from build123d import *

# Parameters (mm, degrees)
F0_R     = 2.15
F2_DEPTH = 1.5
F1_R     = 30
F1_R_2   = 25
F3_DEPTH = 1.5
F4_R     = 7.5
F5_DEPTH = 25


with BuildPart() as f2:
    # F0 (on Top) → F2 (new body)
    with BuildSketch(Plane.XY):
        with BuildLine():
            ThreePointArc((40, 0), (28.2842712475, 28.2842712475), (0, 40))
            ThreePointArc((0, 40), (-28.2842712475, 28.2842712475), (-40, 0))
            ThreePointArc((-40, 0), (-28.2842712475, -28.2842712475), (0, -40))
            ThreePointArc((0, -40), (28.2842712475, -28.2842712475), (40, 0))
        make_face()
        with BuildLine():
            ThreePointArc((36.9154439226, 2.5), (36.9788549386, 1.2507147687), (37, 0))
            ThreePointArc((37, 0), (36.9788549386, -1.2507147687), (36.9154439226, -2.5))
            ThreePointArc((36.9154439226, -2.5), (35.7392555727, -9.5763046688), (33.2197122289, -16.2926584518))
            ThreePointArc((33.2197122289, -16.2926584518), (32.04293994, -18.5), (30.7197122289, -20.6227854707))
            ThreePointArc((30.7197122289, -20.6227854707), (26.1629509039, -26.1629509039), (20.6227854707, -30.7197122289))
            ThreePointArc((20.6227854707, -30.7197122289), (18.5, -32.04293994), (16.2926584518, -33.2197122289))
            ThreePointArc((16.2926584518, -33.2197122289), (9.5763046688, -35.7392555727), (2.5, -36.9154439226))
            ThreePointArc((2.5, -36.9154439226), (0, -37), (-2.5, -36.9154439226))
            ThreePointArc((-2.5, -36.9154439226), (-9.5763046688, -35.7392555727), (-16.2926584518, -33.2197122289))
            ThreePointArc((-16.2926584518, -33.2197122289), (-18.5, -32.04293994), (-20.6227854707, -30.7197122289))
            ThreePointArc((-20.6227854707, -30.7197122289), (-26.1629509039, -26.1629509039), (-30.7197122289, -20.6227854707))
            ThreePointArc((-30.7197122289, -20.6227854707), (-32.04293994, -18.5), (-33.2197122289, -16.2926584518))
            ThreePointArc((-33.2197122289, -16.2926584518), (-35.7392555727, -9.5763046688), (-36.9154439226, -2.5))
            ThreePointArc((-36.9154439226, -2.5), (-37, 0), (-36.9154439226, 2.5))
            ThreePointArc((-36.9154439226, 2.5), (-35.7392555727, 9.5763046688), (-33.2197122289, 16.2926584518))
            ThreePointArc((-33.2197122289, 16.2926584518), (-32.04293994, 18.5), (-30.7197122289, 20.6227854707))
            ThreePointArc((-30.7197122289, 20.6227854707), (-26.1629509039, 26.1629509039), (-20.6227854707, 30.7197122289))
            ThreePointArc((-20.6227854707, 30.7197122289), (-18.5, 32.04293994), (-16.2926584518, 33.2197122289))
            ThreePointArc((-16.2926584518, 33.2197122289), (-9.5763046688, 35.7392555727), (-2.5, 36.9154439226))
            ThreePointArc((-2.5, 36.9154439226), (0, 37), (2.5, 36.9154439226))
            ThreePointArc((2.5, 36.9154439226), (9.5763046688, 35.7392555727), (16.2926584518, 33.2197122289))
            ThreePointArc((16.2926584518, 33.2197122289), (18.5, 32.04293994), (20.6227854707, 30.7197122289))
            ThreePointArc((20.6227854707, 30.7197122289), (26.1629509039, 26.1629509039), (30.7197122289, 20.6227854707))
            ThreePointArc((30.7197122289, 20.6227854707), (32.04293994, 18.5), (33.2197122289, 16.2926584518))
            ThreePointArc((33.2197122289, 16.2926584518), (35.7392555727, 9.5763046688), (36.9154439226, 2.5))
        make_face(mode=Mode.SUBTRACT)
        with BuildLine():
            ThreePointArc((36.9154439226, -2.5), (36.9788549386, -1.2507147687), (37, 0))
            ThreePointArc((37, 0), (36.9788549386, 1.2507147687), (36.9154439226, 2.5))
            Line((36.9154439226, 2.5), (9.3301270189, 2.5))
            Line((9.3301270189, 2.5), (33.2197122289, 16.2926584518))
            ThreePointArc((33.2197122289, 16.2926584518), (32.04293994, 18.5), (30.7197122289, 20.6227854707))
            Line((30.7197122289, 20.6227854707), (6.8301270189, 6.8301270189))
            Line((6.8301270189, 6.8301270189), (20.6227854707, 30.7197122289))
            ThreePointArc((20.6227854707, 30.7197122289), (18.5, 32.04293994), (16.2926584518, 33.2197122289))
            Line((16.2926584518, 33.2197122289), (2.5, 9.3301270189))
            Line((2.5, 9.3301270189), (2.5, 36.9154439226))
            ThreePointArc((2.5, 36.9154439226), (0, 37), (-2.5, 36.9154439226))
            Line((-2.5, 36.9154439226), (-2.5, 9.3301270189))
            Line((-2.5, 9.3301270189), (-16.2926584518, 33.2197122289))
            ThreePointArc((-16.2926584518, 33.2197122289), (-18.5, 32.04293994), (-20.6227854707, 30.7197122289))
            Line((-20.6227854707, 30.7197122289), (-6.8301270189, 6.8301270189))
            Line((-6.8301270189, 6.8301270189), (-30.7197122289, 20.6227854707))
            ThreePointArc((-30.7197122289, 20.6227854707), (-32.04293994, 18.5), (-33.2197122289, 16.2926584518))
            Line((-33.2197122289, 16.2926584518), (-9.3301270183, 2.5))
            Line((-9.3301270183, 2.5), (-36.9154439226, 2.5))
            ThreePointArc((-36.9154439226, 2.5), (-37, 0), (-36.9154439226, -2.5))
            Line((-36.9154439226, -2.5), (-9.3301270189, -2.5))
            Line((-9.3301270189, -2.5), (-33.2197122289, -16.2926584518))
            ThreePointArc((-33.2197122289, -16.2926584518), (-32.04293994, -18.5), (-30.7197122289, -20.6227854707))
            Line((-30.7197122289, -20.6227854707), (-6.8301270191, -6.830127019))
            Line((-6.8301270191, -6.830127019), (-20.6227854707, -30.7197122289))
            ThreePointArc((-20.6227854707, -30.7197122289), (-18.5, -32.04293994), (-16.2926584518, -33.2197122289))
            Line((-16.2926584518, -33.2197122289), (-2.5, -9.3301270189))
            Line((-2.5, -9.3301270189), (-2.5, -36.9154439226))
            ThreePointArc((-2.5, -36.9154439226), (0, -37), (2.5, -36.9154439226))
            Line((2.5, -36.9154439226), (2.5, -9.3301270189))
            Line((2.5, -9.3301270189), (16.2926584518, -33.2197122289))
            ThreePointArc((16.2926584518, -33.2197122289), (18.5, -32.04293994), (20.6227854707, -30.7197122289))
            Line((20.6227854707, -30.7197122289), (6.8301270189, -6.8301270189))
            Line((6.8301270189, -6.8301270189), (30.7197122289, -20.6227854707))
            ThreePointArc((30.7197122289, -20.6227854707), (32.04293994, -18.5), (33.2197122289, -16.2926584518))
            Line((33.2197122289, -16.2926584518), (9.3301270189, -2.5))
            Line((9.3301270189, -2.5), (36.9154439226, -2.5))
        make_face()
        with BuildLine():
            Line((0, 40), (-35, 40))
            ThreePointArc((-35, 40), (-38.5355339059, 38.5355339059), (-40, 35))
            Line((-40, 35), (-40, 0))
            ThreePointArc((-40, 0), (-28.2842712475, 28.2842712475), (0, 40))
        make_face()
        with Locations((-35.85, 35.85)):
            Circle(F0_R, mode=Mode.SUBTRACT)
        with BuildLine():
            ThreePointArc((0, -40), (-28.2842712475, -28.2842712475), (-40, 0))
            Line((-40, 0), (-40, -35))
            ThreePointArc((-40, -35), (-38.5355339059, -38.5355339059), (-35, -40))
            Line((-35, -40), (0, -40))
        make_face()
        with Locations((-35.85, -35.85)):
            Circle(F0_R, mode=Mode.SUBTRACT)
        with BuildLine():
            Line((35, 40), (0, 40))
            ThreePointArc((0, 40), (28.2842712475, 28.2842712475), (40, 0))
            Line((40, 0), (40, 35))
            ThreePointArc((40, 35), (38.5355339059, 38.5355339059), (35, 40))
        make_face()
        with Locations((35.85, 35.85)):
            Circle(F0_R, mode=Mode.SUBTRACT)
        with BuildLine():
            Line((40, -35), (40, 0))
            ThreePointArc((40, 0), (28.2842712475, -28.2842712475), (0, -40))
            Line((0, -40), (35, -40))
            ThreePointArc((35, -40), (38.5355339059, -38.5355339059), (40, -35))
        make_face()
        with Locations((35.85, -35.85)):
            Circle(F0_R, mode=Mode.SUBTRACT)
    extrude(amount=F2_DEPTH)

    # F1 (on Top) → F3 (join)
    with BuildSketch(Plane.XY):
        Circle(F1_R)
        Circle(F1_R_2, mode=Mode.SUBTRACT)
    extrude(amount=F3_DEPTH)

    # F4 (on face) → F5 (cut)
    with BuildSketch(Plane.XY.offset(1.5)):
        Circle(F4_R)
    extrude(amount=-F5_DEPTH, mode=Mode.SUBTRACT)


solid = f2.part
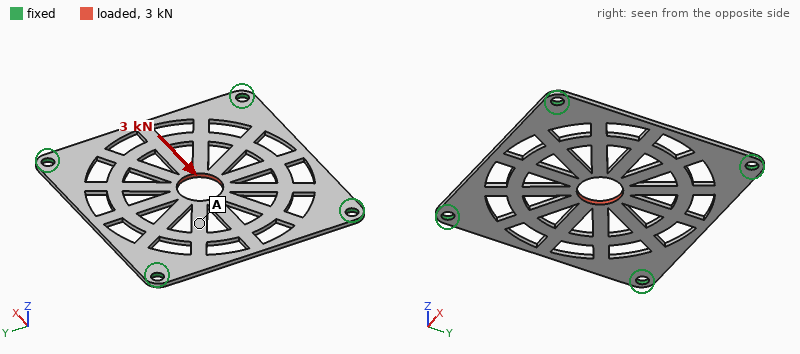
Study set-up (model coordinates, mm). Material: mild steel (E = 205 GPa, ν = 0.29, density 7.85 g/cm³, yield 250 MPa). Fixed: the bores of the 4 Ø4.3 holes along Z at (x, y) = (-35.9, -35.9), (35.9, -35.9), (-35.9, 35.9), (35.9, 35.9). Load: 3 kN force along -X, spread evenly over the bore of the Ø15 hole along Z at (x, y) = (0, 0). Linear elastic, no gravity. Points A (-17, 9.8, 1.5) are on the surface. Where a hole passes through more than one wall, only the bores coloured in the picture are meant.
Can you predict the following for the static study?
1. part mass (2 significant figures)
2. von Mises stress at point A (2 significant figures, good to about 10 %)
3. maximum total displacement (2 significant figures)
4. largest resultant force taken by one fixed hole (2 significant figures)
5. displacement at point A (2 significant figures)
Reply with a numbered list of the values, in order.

1. 51 g
2. 59 MPa
3. 22 µm
4. 850 N
5. 17 µm
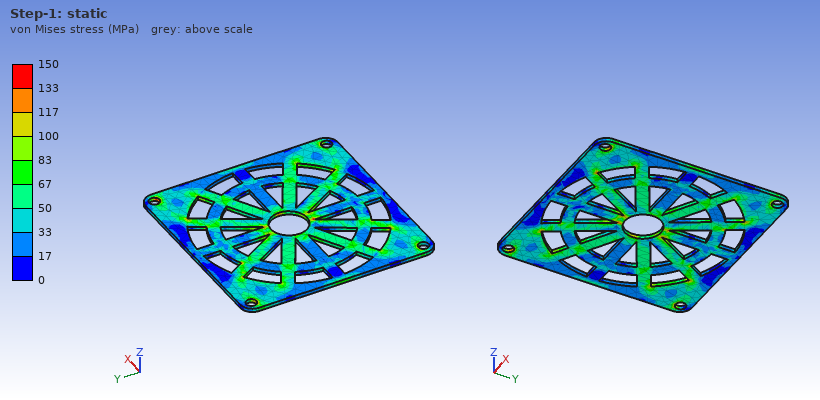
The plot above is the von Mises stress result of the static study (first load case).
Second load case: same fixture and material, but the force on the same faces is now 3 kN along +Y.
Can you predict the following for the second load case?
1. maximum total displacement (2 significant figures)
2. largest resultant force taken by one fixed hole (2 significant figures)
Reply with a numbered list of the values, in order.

1. 22 µm
2. 850 N
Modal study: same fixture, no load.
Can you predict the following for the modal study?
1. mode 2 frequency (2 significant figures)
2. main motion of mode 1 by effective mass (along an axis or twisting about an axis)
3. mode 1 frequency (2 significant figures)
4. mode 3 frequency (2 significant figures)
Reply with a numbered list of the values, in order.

1. 1700 Hz
2. along Z
3. 940 Hz
4. 1700 Hz
